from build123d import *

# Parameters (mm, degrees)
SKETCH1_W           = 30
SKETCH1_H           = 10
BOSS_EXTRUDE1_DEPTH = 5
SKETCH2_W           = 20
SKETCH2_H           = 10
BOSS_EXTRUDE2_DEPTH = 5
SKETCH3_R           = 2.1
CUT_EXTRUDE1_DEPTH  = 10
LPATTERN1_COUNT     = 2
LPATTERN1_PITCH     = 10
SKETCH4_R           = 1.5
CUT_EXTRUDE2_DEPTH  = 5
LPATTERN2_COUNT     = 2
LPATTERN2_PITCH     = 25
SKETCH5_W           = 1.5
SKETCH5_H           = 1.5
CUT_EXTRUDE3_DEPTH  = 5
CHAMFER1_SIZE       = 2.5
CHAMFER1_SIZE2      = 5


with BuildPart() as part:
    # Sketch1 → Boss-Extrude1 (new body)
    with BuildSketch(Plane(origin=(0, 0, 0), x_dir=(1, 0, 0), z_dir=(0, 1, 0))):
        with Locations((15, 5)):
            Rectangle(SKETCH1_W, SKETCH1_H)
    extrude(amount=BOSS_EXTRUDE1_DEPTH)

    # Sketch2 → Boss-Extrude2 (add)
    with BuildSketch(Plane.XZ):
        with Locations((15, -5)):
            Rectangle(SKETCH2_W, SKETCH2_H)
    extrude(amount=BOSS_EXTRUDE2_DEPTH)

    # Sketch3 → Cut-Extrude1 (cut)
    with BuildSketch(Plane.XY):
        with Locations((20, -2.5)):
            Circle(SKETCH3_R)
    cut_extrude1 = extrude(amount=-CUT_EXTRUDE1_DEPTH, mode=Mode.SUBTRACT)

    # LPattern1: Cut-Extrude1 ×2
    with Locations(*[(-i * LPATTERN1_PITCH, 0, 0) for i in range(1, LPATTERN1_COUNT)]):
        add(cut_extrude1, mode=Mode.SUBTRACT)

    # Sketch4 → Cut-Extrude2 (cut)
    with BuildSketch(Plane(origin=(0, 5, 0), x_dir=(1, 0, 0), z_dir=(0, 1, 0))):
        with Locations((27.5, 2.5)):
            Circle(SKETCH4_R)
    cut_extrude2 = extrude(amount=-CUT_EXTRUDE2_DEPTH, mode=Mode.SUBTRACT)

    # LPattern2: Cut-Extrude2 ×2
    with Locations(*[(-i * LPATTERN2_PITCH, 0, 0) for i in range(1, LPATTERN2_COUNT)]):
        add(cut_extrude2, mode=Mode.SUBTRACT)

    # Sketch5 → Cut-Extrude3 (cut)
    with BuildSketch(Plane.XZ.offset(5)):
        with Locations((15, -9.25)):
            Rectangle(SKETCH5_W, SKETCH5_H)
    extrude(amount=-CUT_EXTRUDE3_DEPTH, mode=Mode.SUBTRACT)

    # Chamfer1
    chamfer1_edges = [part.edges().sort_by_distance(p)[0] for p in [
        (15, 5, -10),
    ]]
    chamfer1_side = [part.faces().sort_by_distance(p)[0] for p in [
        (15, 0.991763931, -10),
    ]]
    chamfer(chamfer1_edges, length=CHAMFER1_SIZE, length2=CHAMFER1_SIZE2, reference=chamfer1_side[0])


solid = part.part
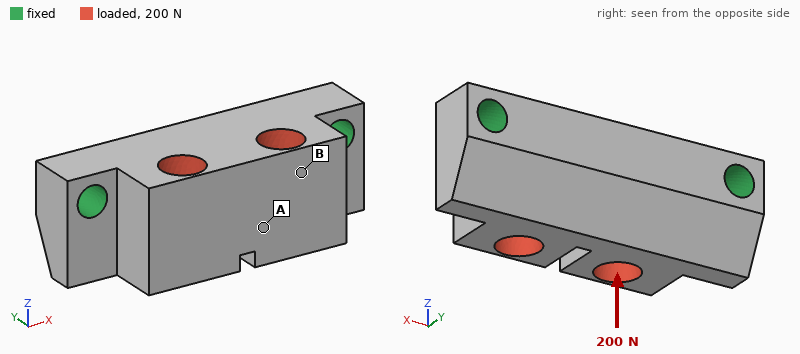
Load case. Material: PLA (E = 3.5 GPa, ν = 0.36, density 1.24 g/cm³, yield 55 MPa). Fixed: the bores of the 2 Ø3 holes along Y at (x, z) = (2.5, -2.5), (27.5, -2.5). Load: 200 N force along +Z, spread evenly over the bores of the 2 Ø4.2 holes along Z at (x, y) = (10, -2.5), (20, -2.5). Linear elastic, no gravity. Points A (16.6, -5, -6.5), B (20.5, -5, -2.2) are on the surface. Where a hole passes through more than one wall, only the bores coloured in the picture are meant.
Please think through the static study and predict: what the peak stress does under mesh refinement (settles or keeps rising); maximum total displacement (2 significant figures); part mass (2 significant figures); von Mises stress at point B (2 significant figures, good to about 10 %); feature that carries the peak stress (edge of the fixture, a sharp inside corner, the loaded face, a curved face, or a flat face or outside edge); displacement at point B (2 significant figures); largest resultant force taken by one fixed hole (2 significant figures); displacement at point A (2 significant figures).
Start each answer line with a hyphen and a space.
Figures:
- keeps rising
- 98 µm
- 2.4 g
- 8.9 MPa
- edge of the fixture
- 75 µm
- 110 N
- 85 µm
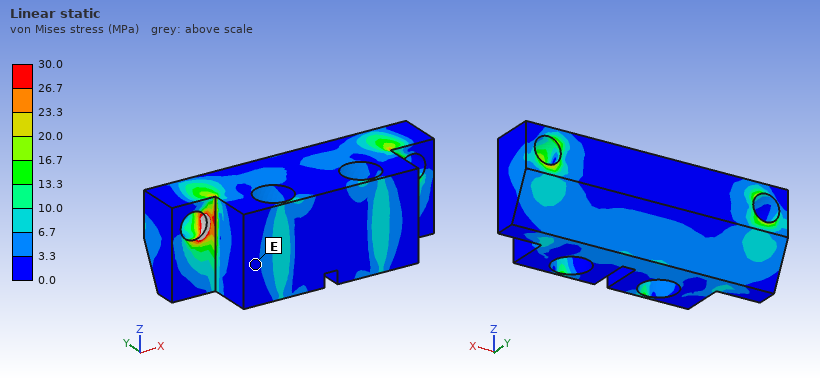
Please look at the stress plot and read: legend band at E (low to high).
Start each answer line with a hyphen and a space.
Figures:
- 0.0 to 3.3 MPa
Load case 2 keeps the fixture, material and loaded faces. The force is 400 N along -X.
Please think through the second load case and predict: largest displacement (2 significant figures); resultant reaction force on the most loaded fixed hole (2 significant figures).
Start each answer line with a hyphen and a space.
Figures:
- 35 µm
- 220 N
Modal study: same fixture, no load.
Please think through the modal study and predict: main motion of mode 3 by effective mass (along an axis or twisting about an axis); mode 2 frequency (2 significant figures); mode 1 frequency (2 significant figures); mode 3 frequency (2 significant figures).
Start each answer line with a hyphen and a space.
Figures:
- along Z
- 11 kHz
- 7700 Hz
- 14 kHz
